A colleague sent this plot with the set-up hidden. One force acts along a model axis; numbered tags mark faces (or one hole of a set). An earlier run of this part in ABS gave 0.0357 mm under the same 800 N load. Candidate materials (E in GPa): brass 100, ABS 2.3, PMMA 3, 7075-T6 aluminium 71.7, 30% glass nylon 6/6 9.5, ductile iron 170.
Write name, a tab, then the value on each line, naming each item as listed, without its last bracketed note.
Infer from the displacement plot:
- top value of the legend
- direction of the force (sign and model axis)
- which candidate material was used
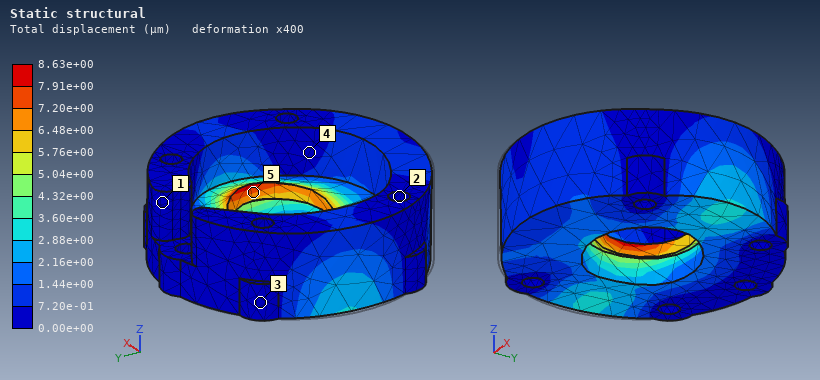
top value of the legend	8.63e+00 µm
direction of the force	+X
which candidate material was used	30% glass nylon 6/6
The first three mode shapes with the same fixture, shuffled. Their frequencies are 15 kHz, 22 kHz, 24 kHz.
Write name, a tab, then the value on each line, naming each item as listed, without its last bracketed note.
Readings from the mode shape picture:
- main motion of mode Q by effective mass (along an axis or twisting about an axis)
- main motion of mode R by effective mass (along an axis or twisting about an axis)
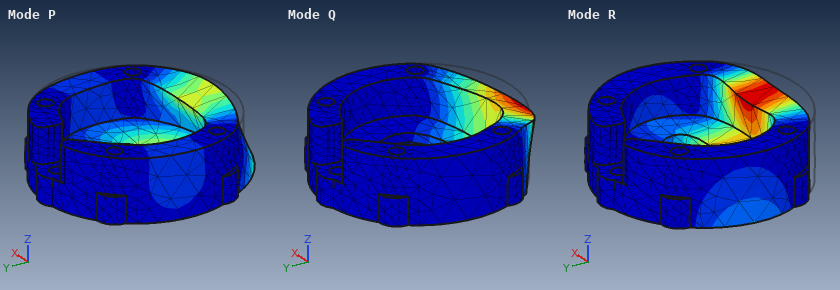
main motion of mode Q by effective mass	along Z
main motion of mode R by effective mass	along Y
